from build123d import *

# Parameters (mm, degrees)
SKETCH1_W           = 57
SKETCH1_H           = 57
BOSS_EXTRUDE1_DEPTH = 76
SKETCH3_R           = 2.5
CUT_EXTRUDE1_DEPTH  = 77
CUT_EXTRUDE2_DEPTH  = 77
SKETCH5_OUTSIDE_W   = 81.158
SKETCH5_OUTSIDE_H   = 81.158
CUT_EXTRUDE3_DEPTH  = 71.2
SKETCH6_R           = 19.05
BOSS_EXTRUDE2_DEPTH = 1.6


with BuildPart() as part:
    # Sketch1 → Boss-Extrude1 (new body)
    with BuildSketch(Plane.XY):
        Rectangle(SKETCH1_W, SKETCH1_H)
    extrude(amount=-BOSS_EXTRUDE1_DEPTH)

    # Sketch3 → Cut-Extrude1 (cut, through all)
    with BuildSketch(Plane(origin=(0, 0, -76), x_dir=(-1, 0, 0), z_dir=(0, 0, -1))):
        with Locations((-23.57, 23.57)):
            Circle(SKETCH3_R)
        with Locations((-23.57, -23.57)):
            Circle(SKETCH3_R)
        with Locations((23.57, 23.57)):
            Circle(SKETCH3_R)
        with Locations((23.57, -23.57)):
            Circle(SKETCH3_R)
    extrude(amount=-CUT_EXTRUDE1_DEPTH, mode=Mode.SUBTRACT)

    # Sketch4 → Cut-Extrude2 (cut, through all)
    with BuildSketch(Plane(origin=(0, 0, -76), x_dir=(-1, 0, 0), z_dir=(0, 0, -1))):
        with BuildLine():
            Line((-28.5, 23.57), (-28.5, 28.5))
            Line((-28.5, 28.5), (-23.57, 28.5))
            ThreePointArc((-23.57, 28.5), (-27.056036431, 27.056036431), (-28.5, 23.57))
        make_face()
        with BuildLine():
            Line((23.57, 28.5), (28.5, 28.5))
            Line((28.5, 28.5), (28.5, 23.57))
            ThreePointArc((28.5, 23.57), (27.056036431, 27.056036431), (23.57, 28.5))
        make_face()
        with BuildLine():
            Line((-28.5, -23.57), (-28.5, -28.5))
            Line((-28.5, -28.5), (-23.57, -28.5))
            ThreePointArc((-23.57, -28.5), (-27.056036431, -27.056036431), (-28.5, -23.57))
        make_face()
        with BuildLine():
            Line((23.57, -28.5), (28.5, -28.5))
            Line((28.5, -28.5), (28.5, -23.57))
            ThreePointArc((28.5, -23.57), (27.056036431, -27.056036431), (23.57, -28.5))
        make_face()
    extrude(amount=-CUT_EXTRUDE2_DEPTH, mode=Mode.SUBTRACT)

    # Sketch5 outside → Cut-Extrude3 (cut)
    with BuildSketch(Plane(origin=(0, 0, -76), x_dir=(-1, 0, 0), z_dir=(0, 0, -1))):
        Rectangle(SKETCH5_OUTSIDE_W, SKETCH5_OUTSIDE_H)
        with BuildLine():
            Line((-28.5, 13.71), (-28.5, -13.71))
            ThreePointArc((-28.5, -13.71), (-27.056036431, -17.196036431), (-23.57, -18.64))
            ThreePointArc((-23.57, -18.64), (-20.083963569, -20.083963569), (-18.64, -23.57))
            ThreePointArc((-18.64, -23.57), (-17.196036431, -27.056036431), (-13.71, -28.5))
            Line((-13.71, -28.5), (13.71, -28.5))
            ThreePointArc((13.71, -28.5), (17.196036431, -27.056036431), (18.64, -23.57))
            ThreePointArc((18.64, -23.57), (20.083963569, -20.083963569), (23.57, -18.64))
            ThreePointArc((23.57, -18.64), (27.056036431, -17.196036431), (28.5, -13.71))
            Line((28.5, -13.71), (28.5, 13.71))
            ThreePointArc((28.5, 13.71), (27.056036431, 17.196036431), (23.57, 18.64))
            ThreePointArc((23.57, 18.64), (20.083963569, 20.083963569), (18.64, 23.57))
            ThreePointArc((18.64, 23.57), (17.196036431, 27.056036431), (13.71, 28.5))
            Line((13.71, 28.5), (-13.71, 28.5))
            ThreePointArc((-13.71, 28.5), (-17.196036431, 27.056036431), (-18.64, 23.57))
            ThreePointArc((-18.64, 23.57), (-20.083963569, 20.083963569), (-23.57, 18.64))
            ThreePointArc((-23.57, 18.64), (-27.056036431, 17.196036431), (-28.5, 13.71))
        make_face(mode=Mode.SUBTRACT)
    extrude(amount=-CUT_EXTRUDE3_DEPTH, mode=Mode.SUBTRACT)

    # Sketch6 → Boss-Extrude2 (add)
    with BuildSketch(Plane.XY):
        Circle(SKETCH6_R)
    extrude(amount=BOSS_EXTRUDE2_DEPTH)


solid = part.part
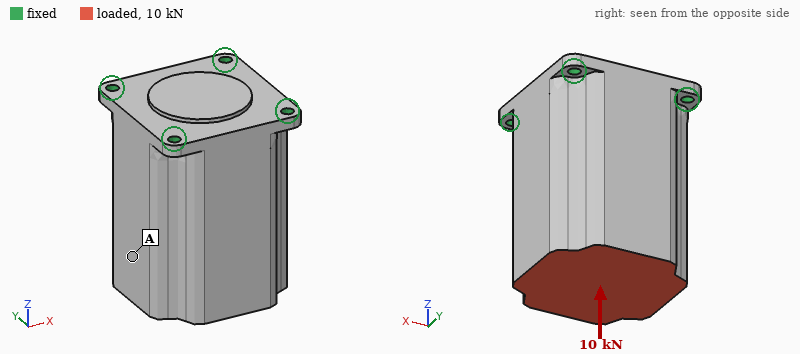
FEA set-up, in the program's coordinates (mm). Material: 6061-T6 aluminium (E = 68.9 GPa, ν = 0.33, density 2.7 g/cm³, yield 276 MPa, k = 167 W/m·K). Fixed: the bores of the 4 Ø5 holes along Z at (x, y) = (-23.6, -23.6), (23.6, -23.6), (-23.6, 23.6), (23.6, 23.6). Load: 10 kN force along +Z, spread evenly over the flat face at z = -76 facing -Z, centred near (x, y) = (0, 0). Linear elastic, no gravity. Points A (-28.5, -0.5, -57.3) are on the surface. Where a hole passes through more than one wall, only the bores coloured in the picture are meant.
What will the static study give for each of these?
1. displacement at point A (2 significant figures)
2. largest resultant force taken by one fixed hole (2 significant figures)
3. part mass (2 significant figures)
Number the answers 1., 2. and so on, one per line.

1. 14 µm
2. 2.7 kN
3. 590 g
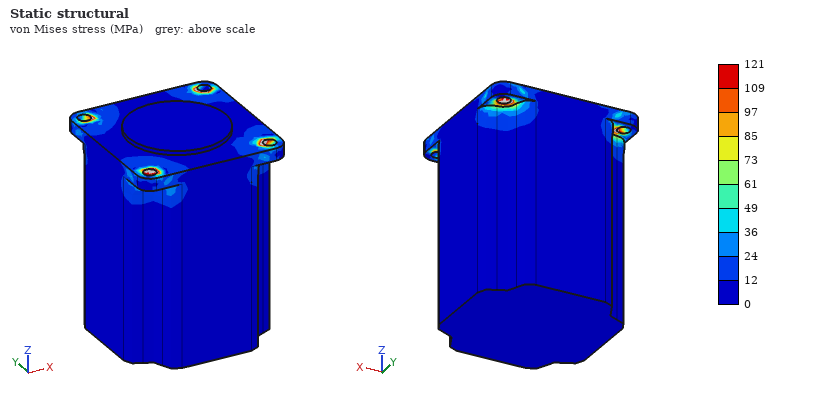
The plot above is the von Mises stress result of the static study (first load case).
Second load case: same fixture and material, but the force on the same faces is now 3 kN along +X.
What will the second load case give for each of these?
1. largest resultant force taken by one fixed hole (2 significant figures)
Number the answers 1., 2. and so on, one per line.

1. 2.7 kN
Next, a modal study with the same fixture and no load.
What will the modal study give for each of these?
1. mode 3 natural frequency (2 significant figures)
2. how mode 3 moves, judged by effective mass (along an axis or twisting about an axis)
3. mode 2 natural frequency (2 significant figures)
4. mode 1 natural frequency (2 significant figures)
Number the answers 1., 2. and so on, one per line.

1. 5800 Hz
2. along Z
3. 2800 Hz
4. 2800 Hz
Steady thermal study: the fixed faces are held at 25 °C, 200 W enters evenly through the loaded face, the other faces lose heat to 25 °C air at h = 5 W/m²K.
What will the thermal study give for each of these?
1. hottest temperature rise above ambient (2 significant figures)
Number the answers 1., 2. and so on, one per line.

1. 56 K
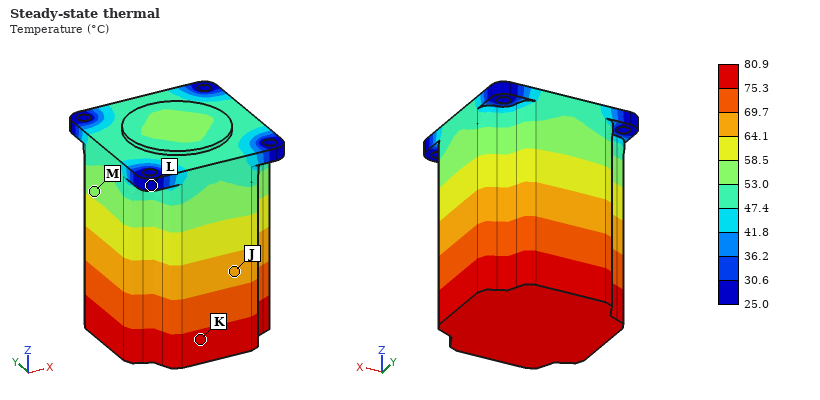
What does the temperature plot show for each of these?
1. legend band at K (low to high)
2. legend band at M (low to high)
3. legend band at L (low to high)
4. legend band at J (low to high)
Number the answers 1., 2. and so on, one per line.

1. 75.3 to 80.9 °C
2. 53.0 to 58.5 °C
3. 25.0 to 30.6 °C
4. 64.1 to 69.7 °C
